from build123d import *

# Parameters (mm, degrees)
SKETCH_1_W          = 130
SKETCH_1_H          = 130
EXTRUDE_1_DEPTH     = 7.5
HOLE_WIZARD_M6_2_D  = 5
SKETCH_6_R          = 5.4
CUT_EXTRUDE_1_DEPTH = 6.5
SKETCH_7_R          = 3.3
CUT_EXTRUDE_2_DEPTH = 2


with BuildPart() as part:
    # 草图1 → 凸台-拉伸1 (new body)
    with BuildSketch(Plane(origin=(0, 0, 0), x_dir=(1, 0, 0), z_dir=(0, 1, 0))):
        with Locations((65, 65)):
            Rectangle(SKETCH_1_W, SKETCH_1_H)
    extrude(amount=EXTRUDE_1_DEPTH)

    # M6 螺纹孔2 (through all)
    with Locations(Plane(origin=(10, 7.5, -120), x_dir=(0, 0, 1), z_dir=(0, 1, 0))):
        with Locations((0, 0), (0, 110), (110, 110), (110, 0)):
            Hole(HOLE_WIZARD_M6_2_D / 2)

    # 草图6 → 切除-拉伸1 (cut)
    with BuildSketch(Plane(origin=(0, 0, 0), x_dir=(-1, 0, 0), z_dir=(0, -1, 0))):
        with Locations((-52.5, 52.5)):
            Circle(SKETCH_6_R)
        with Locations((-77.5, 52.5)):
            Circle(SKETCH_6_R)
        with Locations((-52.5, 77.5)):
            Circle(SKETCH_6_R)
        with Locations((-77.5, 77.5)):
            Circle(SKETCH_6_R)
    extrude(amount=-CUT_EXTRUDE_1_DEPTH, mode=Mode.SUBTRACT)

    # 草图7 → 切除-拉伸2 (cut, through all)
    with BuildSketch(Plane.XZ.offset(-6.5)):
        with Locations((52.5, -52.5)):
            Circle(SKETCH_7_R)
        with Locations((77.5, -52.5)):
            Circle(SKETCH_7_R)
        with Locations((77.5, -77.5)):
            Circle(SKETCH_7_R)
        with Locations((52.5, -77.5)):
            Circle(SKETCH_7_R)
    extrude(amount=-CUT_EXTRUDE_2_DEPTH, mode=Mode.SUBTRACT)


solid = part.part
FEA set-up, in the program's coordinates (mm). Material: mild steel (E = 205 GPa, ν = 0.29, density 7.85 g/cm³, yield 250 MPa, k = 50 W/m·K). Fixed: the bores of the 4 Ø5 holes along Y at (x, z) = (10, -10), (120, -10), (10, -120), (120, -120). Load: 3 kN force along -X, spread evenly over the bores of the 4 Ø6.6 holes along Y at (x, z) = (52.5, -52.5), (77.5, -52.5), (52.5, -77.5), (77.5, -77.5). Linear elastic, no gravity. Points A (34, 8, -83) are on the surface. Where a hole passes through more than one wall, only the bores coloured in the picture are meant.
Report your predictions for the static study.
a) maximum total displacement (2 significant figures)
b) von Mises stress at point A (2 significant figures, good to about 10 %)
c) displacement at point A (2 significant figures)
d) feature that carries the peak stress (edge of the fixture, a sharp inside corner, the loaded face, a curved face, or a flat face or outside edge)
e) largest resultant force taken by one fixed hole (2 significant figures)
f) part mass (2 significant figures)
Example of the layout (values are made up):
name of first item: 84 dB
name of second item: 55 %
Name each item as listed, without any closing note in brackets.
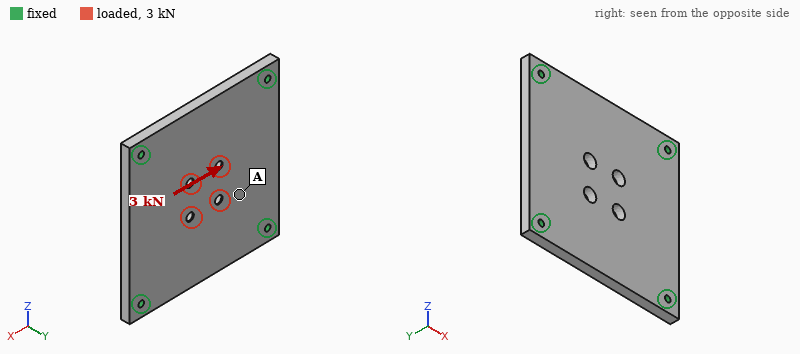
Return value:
maximum total displacement: 3.0 µm
von Mises stress at point A: 4.6 MPa
displacement at point A: 2.0 µm
feature that carries the peak stress: the loaded face
largest resultant force taken by one fixed hole: 840 N
part mass: 970 g
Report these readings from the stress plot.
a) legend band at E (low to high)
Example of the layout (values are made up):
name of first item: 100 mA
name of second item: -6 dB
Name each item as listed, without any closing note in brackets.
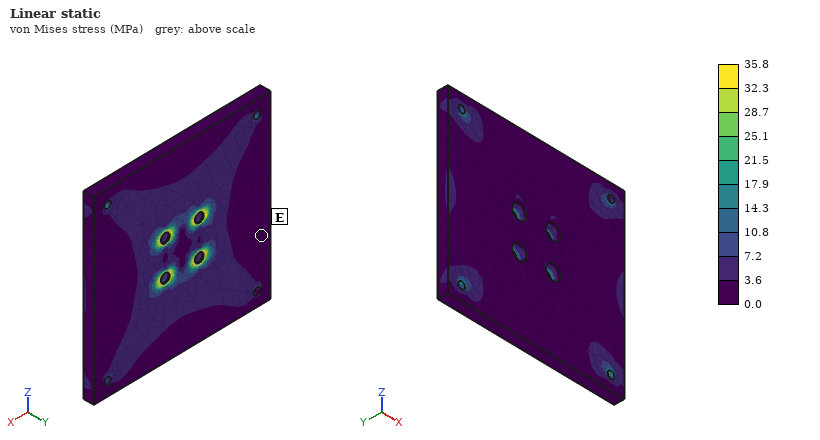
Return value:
legend band at E: 0.0 to 3.6 MPa
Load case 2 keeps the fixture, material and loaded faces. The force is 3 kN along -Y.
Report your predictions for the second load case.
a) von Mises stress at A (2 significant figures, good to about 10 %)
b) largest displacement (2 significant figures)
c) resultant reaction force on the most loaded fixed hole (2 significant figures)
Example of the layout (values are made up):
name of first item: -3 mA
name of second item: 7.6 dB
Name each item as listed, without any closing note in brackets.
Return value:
von Mises stress at A: 25 MPa
largest displacement: 78 µm
resultant reaction force on the most loaded fixed hole: 750 N
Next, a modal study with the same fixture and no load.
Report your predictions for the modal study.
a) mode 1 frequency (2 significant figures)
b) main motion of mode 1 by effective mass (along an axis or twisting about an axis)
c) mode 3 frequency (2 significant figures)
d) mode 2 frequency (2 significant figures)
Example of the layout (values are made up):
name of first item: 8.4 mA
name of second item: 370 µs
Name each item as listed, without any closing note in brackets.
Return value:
mode 1 frequency: 2000 Hz
main motion of mode 1 by effective mass: along Y
mode 3 frequency: 3300 Hz
mode 2 frequency: 3300 Hz
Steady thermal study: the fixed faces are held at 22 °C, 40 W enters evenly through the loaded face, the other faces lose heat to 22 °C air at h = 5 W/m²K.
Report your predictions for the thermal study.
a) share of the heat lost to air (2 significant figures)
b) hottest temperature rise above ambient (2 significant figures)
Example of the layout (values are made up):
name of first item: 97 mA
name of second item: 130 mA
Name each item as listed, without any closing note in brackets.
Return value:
share of the heat lost to air: 9.6 %
hottest temperature rise above ambient: 62 K
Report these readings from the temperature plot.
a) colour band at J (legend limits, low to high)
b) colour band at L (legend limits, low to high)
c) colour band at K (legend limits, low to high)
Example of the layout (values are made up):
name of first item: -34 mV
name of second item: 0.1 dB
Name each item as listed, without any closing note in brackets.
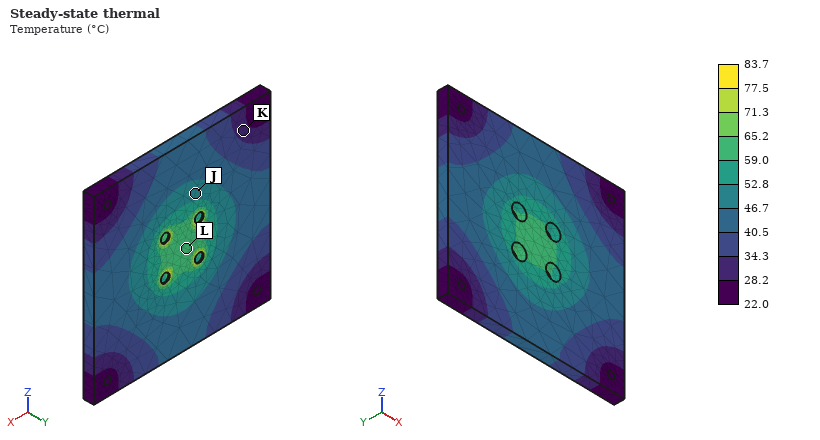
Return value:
colour band at J: 46.7 to 52.8 °C
colour band at L: 59.0 to 65.2 °C
colour band at K: 28.2 to 34.3 °C
